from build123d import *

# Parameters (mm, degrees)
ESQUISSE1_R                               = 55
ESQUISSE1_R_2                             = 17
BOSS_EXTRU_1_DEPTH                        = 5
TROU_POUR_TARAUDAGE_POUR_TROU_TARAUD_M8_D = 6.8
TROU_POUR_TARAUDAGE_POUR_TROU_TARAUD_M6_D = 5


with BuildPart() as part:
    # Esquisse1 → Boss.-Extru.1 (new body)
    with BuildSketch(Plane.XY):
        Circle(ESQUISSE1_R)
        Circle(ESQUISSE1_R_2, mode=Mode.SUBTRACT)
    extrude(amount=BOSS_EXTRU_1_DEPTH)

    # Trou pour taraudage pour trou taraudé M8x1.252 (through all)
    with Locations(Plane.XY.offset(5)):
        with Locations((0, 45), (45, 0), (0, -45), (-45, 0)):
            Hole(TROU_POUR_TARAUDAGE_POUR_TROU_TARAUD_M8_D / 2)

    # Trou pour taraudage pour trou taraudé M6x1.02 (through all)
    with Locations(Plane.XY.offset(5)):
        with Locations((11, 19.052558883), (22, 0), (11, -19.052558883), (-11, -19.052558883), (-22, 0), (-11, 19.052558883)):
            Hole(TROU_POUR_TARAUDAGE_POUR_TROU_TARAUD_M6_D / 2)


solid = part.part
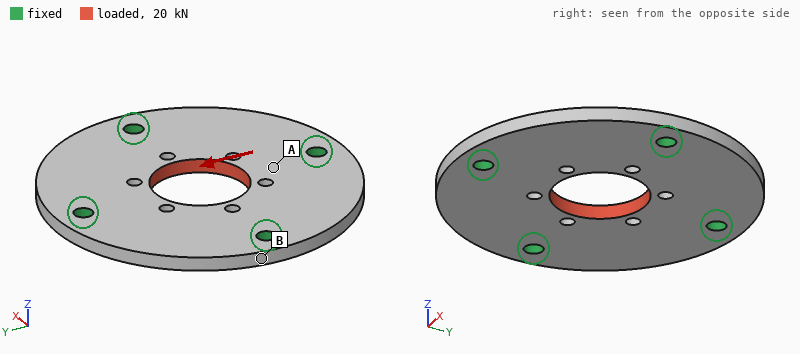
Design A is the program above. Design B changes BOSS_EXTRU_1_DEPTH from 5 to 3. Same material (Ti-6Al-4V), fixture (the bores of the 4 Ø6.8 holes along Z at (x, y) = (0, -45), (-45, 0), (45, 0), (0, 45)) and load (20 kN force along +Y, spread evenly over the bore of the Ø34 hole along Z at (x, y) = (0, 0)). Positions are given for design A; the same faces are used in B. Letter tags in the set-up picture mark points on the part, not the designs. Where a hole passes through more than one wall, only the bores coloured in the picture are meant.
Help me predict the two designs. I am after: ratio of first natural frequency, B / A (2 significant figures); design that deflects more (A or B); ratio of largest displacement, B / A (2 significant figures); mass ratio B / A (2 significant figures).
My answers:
0.64
B
1.7
0.60
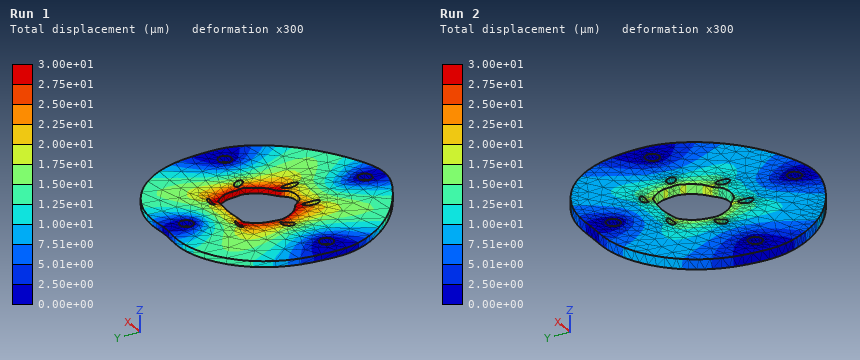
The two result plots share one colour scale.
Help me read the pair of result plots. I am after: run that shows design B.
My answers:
Run 1
